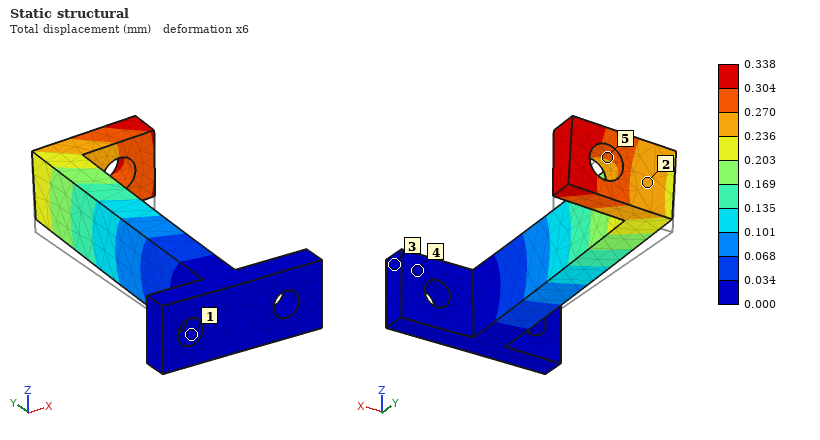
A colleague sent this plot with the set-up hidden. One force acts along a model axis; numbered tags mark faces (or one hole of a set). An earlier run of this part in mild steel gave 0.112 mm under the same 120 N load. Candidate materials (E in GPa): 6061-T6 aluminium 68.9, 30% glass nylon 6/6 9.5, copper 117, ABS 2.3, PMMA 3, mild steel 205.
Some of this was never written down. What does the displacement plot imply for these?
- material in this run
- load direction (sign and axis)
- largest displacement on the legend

6061-T6 aluminium
+Z
0.338 mm
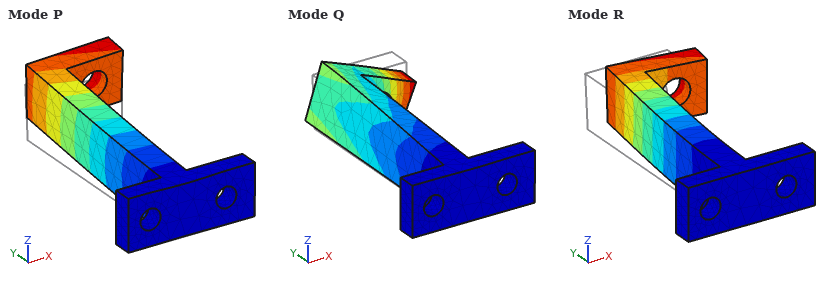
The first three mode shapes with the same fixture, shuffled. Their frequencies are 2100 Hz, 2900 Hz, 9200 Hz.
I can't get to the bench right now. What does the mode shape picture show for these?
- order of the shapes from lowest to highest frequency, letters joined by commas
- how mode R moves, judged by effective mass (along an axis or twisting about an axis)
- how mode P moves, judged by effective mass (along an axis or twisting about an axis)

R, P, Q
along X
along Z
